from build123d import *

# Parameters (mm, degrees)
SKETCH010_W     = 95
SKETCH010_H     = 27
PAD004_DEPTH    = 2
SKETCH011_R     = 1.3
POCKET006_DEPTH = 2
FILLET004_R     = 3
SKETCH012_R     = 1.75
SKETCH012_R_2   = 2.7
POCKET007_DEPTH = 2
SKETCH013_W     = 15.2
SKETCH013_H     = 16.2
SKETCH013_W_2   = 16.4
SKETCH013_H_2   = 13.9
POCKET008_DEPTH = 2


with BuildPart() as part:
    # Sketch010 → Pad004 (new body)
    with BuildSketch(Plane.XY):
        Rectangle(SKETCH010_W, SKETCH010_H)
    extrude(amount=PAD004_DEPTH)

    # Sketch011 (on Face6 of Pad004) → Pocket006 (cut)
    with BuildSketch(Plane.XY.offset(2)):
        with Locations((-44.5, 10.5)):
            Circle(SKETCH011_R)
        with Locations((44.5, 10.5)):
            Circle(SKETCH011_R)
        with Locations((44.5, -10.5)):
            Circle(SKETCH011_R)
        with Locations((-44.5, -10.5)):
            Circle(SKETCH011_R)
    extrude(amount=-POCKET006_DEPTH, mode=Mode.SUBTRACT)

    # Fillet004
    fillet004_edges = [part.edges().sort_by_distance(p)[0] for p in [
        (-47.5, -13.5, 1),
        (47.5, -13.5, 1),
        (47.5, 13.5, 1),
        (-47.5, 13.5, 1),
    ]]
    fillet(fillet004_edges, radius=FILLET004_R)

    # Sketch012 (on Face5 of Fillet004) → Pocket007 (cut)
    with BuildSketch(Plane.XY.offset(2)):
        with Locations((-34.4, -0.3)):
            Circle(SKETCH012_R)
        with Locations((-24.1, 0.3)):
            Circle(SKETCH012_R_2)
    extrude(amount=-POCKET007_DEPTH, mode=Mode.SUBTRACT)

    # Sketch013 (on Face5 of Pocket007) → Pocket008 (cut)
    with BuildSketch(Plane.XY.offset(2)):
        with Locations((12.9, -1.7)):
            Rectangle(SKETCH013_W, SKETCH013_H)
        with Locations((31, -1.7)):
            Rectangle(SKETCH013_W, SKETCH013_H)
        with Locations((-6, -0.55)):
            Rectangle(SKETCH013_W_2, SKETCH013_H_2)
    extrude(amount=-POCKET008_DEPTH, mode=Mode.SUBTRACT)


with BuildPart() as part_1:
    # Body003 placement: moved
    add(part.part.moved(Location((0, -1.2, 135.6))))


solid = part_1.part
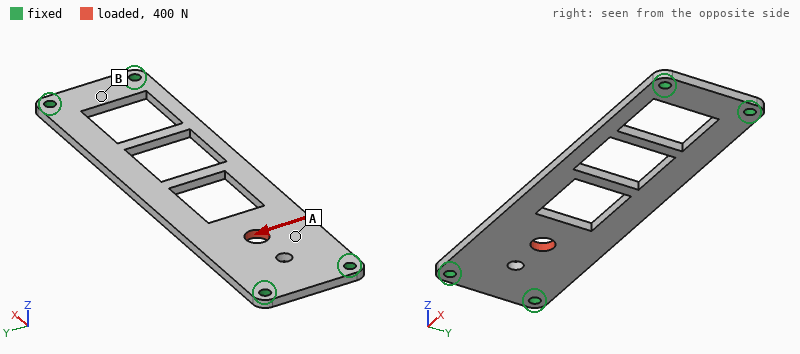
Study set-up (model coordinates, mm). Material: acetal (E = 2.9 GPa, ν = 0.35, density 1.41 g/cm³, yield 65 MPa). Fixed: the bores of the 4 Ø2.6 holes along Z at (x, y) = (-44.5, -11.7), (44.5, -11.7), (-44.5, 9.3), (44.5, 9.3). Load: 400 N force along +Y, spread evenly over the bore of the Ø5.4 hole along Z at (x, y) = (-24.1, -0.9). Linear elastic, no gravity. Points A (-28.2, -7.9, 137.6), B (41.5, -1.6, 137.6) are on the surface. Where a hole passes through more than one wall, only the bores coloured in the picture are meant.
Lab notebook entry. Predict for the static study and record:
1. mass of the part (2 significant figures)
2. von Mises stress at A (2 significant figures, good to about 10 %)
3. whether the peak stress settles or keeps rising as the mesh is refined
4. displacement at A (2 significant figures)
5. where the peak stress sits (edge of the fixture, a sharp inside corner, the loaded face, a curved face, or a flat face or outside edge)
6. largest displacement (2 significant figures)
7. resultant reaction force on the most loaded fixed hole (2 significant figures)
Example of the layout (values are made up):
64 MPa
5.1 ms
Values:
5.0 g
12 MPa
keeps rising
0.22 mm
edge of the fixture
0.36 mm
370 N
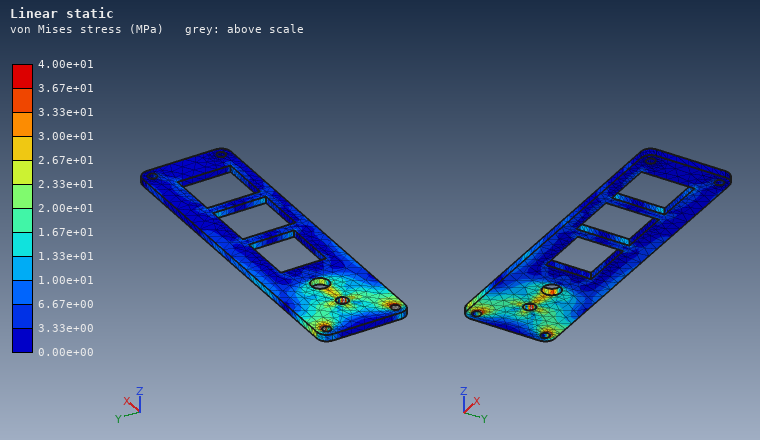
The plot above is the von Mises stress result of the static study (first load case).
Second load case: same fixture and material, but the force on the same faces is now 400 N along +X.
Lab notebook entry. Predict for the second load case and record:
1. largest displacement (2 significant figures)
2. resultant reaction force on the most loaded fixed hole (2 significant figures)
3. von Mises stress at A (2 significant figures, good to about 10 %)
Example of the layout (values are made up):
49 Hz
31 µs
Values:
97 µm
180 N
7.6 MPa
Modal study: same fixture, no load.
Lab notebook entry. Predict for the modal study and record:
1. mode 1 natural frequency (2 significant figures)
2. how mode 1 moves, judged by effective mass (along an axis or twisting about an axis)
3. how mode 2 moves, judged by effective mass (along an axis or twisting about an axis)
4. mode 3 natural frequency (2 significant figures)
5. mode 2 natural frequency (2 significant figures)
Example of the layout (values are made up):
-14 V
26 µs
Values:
370 Hz
along Z
twisting about X
970 Hz
740 Hz
